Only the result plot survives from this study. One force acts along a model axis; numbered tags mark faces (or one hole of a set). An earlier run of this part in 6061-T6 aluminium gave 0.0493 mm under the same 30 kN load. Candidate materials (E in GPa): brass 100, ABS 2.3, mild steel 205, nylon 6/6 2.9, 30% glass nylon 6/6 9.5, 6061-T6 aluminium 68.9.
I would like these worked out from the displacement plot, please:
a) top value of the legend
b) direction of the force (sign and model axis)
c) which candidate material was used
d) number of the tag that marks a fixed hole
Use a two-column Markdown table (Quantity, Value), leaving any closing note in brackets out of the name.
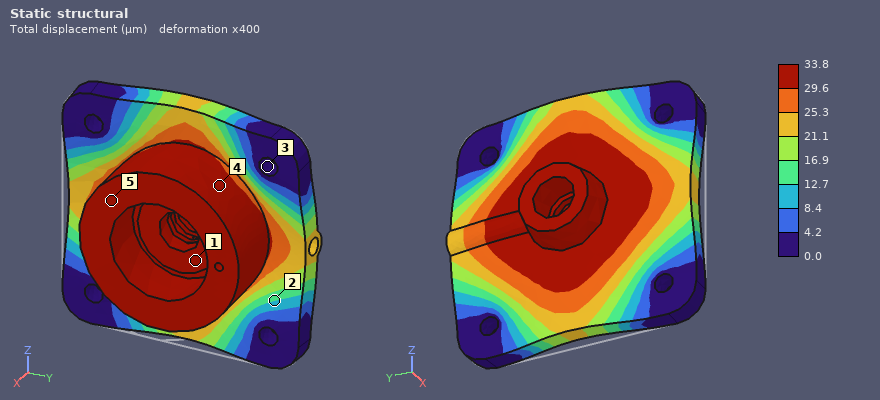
| Quantity | Value |
|---|---|
| top value of the legend | 33.8 µm |
| direction of the force | -X |
| which candidate material was used | brass |
| number of the tag that marks a fixed hole | 3 |
